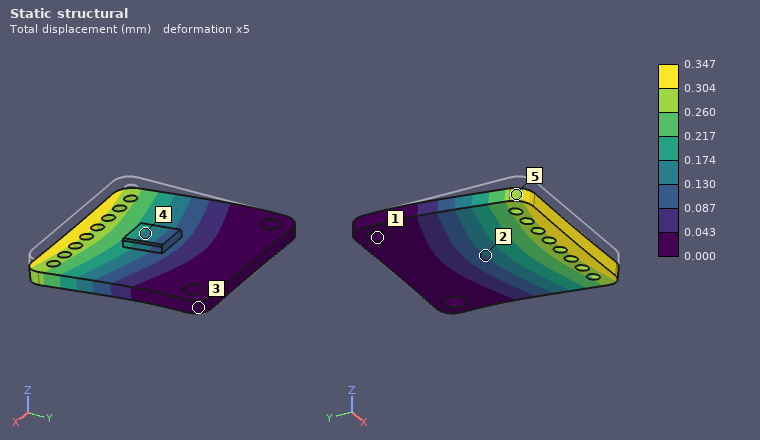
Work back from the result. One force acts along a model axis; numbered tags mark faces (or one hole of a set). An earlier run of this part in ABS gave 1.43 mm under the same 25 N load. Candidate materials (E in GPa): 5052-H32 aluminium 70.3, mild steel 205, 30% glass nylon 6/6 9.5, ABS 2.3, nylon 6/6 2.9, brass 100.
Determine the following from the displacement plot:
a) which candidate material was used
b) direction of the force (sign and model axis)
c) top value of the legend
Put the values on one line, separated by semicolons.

30% glass nylon 6/6; -Z; 0.347 mm
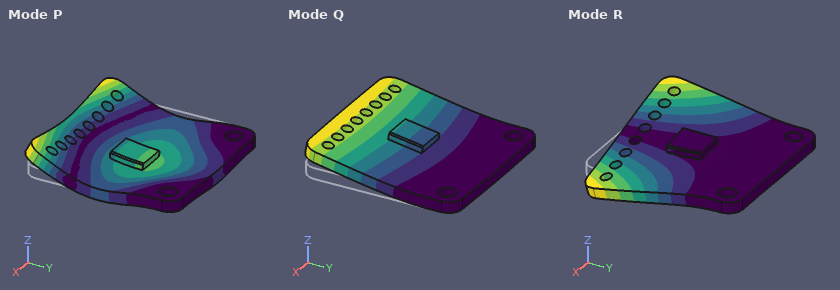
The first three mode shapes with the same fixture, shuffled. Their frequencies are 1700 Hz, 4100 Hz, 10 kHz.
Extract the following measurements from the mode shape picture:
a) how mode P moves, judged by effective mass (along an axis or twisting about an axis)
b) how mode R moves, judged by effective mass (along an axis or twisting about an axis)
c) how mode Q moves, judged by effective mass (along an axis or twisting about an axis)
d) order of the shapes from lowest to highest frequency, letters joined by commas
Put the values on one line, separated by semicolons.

along Z; twisting about Y; along Z; Q, R, P
